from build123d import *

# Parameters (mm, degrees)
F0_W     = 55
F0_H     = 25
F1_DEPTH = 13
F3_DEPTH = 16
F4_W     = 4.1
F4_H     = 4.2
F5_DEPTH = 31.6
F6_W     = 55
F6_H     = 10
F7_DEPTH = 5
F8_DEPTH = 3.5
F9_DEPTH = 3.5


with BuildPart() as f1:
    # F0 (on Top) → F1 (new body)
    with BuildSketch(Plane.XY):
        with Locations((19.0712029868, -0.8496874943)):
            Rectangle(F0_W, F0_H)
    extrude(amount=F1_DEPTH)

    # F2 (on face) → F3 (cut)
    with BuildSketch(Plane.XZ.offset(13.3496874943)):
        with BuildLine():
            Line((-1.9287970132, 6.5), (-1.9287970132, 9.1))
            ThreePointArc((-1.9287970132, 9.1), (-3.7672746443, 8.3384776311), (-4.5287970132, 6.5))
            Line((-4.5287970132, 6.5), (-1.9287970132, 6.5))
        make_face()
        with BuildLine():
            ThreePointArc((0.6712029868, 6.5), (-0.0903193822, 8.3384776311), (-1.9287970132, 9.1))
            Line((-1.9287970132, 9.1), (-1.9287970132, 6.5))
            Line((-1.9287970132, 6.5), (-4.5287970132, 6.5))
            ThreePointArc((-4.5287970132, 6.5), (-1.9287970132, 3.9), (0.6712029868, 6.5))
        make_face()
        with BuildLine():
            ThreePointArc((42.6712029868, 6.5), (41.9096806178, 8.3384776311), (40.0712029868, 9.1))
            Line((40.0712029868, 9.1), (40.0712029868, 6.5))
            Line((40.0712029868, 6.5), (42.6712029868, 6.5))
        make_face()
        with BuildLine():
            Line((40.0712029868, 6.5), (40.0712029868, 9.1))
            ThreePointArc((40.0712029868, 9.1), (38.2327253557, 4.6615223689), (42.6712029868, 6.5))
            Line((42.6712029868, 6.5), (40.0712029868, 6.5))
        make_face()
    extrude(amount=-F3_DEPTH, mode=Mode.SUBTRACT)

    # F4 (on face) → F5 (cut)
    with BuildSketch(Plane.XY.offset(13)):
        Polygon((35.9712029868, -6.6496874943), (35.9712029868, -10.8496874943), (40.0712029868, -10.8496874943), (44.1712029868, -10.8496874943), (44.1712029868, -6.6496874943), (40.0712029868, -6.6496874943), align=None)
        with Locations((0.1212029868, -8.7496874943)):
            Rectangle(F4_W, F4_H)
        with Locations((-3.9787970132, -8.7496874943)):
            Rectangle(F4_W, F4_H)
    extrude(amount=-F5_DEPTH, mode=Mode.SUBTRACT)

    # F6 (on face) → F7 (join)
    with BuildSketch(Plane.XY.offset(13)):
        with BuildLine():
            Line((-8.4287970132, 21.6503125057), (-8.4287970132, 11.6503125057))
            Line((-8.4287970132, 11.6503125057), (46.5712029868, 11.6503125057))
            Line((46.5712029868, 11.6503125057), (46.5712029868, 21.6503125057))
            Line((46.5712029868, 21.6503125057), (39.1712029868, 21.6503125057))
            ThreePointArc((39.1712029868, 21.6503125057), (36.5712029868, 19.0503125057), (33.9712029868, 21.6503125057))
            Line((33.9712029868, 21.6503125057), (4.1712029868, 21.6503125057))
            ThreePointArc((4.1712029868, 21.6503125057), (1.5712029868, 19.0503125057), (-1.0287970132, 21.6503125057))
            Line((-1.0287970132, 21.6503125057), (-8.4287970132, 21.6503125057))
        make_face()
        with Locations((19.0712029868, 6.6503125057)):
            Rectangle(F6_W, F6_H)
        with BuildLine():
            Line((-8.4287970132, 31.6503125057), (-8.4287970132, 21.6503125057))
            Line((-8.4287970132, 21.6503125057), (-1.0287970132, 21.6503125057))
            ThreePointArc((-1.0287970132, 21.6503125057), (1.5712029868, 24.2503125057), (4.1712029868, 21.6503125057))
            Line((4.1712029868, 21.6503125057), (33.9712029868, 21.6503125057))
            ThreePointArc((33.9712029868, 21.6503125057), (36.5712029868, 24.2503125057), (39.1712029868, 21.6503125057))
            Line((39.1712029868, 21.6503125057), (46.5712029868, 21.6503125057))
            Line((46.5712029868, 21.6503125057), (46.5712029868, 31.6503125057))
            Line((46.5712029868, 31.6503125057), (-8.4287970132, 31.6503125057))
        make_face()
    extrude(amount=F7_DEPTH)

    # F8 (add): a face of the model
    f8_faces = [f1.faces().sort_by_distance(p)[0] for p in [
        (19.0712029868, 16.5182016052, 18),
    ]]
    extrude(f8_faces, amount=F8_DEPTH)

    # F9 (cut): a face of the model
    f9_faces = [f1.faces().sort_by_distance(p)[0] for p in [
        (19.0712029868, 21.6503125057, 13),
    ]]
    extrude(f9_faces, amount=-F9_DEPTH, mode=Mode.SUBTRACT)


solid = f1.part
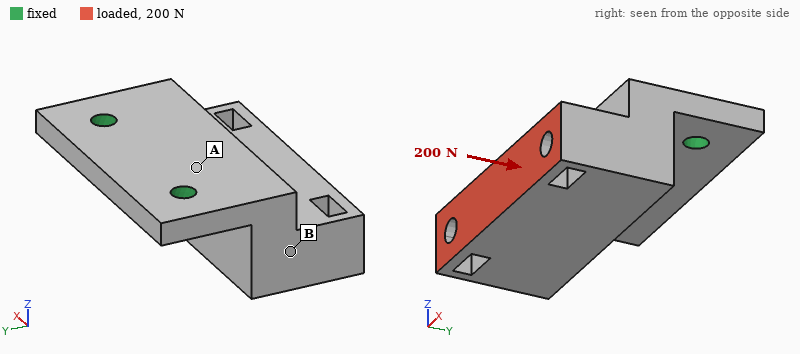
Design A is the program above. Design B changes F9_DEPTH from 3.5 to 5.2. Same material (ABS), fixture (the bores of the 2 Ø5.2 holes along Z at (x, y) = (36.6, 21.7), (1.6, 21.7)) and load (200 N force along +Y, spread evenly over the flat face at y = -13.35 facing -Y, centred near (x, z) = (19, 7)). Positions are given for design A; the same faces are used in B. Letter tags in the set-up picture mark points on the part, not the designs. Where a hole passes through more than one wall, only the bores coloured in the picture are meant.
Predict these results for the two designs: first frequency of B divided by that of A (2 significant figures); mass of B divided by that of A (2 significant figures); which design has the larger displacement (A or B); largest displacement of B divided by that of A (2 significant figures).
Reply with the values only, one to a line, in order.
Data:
0.56
0.93
B
3.2
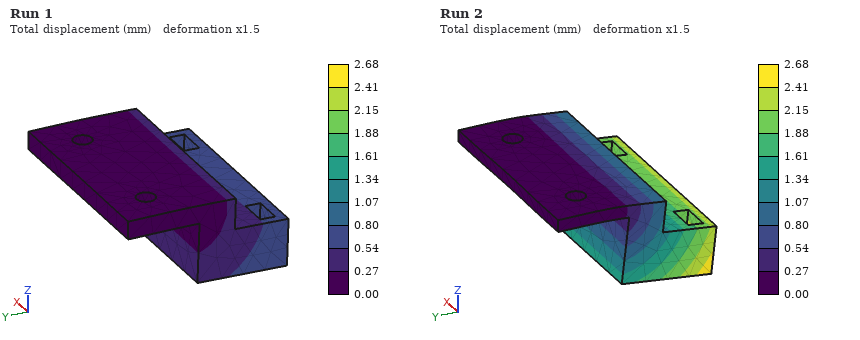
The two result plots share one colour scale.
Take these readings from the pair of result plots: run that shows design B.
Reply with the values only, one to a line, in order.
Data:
Run 2
